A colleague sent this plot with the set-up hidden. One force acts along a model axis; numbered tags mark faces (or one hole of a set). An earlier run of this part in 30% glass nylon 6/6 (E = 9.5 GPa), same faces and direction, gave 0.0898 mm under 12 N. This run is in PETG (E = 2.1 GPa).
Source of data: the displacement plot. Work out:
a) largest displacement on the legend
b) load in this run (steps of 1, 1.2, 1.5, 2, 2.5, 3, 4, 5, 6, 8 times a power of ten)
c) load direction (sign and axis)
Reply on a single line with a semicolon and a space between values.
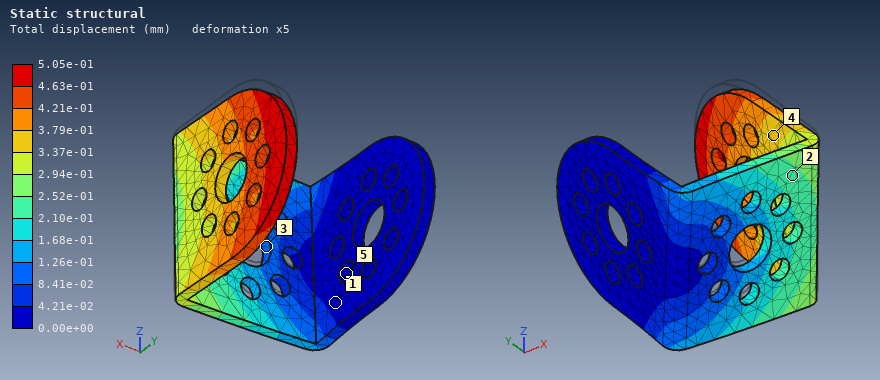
5.05e-01 mm; 15 N; -Z
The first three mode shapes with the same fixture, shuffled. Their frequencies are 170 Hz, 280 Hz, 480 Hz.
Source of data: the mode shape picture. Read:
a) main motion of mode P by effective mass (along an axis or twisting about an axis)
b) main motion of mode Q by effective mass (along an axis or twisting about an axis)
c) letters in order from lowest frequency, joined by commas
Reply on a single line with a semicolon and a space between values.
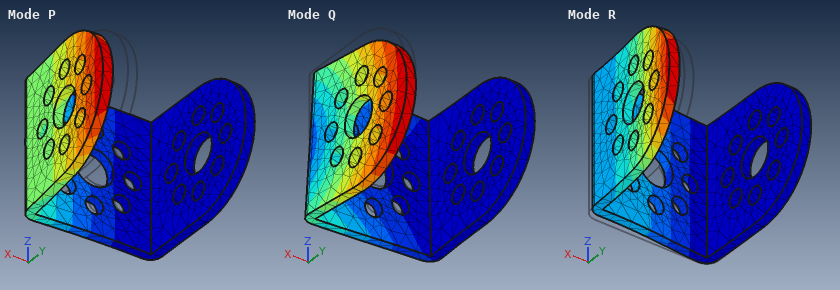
along Y; along Z; P, Q, R
